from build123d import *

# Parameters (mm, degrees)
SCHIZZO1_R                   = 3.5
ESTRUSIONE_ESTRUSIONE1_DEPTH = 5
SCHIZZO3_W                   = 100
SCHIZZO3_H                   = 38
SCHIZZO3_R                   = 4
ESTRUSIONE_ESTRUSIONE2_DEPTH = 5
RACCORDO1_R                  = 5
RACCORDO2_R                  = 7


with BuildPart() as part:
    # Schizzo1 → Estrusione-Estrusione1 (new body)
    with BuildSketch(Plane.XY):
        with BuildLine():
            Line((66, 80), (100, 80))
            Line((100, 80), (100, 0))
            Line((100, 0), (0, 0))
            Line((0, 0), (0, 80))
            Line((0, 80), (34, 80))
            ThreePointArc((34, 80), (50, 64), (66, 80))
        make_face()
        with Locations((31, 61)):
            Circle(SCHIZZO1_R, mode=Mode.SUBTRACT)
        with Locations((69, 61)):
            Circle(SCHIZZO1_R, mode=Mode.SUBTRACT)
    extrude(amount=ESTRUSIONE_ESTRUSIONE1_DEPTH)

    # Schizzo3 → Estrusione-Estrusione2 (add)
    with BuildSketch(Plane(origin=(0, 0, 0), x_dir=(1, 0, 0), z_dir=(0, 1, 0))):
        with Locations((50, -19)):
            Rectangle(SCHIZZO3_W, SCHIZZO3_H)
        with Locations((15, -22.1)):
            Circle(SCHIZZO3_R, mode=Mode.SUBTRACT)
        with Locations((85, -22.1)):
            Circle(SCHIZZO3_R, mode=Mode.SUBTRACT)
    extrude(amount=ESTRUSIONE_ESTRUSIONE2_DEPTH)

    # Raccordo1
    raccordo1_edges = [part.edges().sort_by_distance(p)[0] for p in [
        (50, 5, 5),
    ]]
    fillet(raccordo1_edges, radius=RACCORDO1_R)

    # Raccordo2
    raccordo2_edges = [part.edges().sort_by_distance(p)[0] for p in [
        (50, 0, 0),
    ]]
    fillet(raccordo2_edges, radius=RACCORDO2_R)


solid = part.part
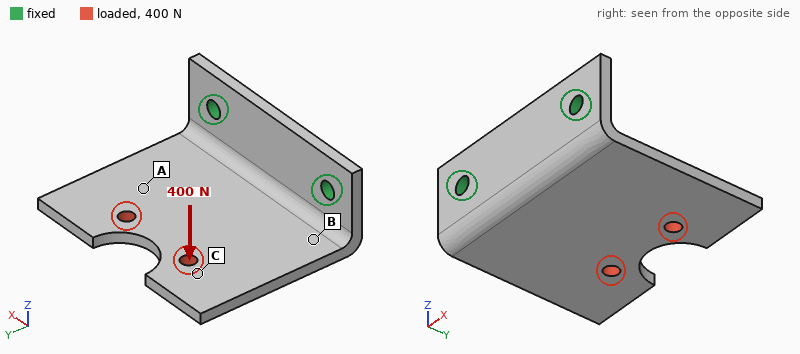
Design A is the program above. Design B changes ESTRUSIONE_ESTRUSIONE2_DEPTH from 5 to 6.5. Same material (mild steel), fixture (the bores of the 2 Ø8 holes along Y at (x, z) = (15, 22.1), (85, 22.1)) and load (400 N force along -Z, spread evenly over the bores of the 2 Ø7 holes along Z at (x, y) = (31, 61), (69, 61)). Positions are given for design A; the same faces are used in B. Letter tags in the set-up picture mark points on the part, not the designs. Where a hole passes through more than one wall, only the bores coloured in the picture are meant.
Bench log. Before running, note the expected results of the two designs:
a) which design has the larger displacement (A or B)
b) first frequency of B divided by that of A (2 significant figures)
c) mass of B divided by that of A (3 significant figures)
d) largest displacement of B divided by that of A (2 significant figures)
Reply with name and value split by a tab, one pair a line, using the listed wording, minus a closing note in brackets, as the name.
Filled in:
which design has the larger displacement	A
first frequency of B divided by that of A	1.2
mass of B divided by that of A	1.09
largest displacement of B divided by that of A	0.71
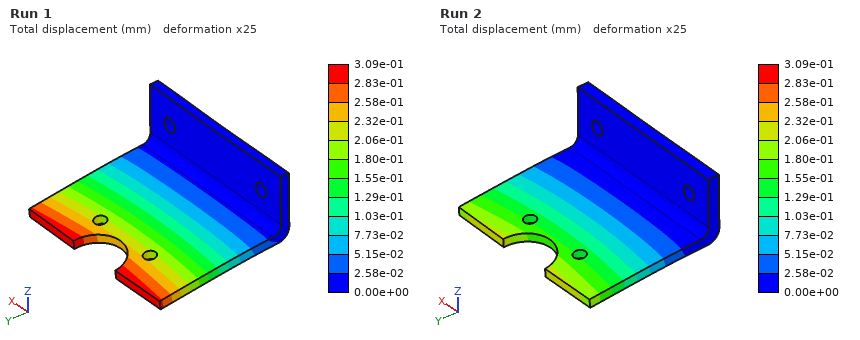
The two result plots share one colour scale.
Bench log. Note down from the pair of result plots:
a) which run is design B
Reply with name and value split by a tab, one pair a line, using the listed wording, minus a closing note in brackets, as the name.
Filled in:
which run is design B	Run 2
